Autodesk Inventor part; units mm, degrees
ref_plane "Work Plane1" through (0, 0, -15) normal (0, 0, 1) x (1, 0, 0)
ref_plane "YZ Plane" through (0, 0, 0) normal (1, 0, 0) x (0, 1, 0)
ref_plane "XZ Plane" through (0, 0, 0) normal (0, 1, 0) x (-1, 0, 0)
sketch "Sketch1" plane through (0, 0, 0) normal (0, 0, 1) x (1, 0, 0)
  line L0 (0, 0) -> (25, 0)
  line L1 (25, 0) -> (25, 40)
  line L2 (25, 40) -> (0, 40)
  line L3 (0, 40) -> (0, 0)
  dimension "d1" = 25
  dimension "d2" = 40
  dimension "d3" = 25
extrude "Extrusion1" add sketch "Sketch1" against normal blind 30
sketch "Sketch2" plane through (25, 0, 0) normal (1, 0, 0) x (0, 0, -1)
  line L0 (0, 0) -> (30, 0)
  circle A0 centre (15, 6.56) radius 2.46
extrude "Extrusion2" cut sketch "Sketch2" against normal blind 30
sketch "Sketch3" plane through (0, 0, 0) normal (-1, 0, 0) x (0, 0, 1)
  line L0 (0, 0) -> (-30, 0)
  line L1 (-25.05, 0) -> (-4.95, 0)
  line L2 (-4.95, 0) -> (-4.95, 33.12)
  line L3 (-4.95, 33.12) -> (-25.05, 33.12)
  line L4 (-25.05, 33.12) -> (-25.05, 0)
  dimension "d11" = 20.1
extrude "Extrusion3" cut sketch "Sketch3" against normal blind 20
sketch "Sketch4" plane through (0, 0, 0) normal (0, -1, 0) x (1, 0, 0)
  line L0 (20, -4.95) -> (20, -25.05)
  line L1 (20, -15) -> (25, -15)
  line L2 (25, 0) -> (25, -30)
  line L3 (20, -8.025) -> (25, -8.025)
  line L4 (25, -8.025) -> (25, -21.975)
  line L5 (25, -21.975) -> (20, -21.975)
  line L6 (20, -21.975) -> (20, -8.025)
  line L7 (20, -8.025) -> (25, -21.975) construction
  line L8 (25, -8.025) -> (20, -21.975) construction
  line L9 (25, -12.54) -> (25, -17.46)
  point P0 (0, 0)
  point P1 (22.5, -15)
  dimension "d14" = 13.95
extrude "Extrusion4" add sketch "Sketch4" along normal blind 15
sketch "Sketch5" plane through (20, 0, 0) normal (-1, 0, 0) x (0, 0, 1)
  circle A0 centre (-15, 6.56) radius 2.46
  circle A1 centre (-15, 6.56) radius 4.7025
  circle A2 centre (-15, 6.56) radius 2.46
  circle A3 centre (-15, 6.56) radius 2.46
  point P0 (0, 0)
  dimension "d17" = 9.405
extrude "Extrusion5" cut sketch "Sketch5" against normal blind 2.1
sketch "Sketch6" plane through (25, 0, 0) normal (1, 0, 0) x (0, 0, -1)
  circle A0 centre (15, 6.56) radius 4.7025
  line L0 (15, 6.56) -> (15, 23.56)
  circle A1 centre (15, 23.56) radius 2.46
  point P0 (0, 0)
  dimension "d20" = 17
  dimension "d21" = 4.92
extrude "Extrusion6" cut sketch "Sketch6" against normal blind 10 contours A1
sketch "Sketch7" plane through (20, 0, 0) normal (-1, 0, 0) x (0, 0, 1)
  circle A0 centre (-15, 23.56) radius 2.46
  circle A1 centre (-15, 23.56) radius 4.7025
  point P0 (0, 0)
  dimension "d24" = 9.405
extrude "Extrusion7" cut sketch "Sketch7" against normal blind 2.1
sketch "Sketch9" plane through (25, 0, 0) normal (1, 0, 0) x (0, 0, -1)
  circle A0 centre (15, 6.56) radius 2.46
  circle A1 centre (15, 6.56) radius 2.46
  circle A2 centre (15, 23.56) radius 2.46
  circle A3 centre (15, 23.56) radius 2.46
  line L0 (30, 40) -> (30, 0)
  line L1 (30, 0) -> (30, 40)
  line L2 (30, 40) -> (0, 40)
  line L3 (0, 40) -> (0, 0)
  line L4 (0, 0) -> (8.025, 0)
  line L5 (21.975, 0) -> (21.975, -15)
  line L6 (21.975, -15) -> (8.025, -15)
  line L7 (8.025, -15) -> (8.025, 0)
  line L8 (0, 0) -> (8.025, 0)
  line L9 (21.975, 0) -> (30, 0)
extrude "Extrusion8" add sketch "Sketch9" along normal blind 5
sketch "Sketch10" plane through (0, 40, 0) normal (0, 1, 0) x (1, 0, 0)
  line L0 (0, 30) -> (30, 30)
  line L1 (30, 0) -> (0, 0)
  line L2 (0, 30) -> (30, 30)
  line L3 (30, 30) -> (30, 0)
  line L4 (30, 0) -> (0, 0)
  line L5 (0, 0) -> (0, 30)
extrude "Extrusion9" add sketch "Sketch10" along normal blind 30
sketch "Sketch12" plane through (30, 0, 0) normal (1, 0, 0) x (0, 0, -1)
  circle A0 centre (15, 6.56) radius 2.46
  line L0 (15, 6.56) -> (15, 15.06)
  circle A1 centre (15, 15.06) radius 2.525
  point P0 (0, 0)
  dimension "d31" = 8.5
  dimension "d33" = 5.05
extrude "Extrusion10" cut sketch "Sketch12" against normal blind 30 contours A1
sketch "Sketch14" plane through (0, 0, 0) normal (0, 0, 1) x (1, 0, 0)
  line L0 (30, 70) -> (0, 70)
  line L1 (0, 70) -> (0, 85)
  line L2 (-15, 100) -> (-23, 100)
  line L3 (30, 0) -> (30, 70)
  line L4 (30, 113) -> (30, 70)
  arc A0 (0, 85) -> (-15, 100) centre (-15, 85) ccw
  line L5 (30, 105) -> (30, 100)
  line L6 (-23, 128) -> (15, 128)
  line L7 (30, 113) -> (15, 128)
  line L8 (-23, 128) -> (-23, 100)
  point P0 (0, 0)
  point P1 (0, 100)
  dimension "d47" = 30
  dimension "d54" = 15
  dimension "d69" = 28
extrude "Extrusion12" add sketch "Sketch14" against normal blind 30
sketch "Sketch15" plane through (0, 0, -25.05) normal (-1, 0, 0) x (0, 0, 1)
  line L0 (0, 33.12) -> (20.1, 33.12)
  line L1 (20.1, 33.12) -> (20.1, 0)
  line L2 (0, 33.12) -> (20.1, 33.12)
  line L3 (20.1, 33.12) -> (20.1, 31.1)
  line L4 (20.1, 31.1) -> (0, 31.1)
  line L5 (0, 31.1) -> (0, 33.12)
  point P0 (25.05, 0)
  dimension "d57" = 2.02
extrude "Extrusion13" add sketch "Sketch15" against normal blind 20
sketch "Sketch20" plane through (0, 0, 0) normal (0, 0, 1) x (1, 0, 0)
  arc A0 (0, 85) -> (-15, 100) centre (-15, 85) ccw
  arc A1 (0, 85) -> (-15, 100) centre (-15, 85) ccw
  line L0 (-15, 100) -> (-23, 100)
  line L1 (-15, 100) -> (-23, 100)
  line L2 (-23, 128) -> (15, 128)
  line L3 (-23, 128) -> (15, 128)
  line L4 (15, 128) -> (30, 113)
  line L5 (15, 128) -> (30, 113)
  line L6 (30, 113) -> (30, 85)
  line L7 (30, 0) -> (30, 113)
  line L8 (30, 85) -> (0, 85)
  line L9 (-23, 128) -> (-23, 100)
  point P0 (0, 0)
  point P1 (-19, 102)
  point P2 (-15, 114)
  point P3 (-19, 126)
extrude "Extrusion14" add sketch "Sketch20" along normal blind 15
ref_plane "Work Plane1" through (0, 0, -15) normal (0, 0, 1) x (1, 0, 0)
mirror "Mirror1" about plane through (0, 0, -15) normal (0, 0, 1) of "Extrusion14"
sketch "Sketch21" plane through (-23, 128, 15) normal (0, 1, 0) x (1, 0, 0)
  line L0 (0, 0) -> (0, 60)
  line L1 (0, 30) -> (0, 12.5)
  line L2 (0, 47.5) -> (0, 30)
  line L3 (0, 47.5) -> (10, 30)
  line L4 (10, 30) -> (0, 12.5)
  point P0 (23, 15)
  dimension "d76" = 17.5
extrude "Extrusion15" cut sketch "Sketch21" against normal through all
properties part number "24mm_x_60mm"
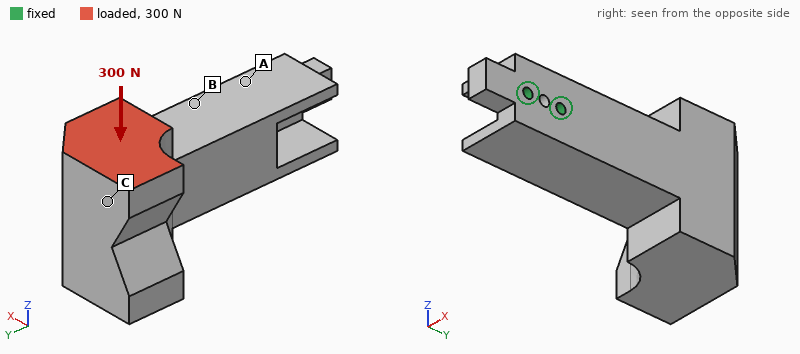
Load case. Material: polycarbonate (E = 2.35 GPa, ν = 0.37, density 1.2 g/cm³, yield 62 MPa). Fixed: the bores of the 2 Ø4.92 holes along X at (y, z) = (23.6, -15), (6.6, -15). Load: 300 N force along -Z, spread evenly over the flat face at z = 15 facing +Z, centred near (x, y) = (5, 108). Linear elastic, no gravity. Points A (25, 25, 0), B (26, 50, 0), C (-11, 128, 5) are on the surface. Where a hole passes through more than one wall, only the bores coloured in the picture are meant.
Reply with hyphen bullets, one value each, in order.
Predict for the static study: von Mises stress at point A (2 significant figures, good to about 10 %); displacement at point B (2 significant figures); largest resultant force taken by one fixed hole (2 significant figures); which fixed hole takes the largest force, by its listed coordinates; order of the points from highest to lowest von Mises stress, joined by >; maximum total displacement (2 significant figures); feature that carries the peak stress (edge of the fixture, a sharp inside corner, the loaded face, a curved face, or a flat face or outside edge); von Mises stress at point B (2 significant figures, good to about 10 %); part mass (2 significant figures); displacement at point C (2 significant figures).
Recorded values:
- 11 MPa
- 0.38 mm
- 1.4 kN
- (23.6, -15)
- A > B > C
- 1.9 mm
- edge of the fixture
- 4.3 MPa
- 210 g
- 1.8 mm
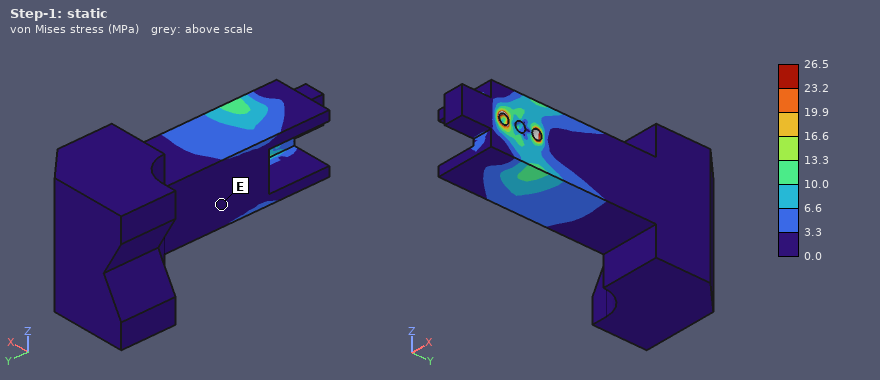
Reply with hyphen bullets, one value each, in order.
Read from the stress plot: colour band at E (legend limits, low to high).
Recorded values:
- 0.0 to 3.3 MPa
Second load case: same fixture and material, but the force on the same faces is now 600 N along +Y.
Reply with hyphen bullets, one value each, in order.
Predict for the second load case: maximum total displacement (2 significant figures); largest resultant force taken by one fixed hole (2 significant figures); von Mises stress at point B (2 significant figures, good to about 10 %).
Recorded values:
- 1.9 mm
- 980 N
- 4.6 MPa
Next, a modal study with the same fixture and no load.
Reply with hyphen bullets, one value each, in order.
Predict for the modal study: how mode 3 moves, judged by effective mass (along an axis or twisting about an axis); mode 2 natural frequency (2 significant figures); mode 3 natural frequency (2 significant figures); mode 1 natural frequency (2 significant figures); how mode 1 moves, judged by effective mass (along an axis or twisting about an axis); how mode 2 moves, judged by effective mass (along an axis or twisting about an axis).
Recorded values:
- twisting about Y
- 200 Hz
- 430 Hz
- 170 Hz
- along X
- along Z
